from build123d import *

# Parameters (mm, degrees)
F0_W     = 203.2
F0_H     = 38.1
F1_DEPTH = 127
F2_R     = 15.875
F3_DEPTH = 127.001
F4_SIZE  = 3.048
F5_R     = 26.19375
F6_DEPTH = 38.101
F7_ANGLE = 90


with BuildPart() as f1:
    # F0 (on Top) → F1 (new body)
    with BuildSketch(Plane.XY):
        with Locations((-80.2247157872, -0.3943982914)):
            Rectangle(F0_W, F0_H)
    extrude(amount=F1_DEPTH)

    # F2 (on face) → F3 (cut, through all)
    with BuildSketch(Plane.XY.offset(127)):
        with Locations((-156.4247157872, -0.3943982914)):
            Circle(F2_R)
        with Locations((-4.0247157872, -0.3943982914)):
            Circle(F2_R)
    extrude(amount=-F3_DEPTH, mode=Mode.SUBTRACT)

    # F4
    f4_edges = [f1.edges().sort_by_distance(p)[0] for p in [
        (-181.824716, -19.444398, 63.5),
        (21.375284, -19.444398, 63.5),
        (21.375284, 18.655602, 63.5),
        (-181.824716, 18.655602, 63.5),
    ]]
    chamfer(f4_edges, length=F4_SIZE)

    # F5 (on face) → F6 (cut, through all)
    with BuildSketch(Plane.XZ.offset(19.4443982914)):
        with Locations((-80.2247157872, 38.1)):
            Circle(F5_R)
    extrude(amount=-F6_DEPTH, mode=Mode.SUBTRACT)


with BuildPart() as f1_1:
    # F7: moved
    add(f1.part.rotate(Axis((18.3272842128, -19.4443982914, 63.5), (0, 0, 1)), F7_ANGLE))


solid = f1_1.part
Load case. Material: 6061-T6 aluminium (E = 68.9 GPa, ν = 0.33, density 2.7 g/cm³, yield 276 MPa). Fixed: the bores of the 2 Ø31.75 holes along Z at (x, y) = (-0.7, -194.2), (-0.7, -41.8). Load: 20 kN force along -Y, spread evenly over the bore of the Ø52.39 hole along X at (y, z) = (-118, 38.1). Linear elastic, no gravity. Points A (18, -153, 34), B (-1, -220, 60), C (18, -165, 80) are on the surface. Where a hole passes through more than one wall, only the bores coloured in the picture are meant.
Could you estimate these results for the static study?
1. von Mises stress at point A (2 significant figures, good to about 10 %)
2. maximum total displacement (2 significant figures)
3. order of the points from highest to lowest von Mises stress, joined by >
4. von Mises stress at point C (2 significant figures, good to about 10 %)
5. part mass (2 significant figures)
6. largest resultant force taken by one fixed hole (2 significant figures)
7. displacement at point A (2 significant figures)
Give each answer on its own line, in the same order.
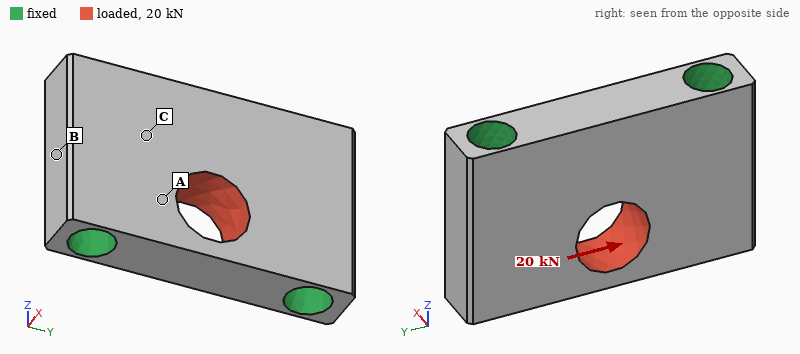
3.2 MPa
3.4 µm
A > C > B
1.4 MPa
1.9 kg
10 kN
1.3 µm
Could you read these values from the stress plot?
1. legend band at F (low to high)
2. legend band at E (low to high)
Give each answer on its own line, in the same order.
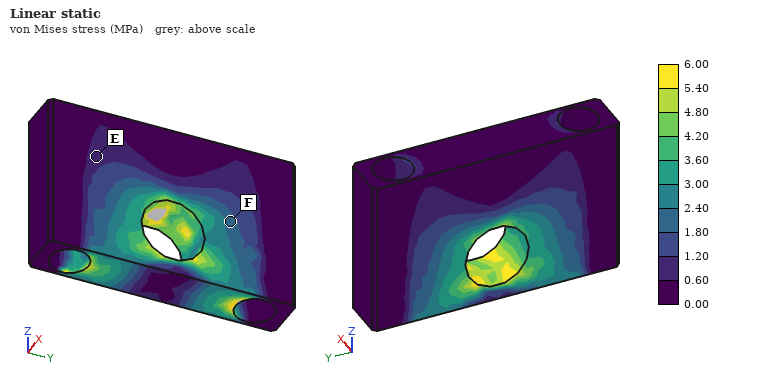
1.80 to 2.40 MPa
0.60 to 1.20 MPa
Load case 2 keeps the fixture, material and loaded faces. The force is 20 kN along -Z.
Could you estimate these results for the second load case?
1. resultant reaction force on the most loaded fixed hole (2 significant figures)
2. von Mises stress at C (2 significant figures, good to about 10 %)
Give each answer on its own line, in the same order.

10 kN
3.5 MPa
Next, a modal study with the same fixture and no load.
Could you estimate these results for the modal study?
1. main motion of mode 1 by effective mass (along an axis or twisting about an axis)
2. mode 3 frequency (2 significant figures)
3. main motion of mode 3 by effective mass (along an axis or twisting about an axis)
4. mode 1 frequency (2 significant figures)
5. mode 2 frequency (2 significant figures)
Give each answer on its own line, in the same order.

along X
12 kHz
along Z
8300 Hz
9700 Hz
